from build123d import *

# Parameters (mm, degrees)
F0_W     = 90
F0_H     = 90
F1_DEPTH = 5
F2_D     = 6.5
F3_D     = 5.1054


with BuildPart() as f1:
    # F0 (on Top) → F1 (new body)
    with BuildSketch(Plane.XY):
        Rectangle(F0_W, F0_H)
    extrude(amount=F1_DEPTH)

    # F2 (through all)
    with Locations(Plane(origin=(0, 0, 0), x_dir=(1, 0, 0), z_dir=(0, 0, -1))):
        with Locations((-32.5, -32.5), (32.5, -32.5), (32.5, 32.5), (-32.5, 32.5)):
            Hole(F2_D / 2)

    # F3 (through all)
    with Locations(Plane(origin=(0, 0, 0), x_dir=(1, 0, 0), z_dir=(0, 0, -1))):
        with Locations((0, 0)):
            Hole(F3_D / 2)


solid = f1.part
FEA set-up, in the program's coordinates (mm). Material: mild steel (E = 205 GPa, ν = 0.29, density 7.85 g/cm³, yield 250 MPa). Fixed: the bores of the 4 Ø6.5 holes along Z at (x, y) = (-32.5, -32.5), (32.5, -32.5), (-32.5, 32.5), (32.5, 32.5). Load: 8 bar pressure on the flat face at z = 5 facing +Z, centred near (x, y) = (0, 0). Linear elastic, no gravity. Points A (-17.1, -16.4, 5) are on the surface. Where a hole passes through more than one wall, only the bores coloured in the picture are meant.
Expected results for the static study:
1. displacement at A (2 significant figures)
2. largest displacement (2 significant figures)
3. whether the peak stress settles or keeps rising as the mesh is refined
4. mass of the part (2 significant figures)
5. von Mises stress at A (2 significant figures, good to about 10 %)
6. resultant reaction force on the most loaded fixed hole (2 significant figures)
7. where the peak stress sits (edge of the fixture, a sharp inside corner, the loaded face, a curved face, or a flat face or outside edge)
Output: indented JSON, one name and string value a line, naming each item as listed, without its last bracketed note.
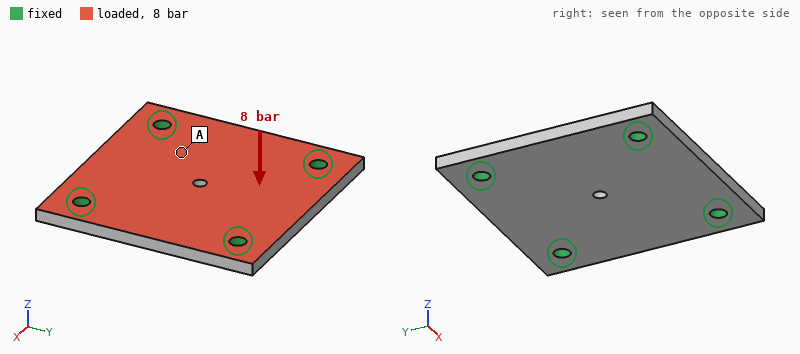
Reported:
{
  "displacement at A": "24 µm",
  "largest displacement": "40 µm",
  "whether the peak stress settles or keeps rising as the mesh is refined": "keeps rising",
  "mass of the part": "310 g",
  "von Mises stress at A": "17 MPa",
  "resultant reaction force on the most loaded fixed hole": "1.6 kN",
  "where the peak stress sits": "edge of the fixture"
}
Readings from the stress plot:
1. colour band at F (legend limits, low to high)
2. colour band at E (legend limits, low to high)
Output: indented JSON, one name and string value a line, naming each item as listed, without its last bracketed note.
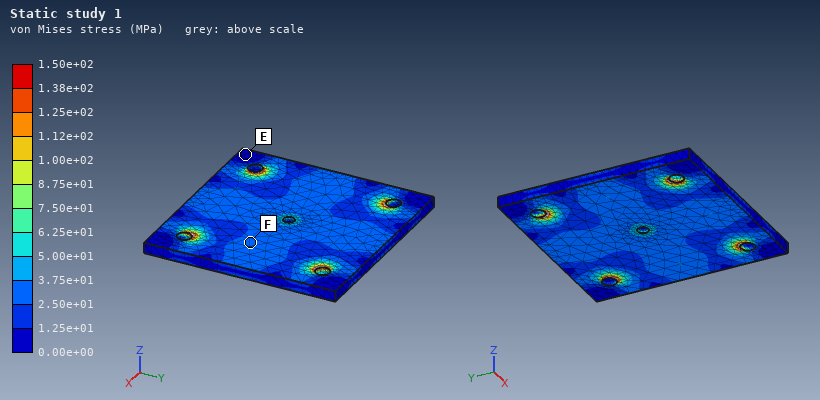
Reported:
{
  "colour band at F": "2.50e+01 to 3.75e+01 MPa",
  "colour band at E": "0.00e+00 to 1.25e+01 MPa"
}
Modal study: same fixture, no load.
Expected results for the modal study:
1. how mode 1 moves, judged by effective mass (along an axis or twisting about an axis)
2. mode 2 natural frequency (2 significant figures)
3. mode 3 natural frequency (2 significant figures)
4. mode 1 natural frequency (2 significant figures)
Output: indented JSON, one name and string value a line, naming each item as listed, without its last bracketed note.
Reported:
{
  "how mode 1 moves, judged by effective mass": "along Z",
  "mode 2 natural frequency": "6800 Hz",
  "mode 3 natural frequency": "6800 Hz",
  "mode 1 natural frequency": "4500 Hz"
}
